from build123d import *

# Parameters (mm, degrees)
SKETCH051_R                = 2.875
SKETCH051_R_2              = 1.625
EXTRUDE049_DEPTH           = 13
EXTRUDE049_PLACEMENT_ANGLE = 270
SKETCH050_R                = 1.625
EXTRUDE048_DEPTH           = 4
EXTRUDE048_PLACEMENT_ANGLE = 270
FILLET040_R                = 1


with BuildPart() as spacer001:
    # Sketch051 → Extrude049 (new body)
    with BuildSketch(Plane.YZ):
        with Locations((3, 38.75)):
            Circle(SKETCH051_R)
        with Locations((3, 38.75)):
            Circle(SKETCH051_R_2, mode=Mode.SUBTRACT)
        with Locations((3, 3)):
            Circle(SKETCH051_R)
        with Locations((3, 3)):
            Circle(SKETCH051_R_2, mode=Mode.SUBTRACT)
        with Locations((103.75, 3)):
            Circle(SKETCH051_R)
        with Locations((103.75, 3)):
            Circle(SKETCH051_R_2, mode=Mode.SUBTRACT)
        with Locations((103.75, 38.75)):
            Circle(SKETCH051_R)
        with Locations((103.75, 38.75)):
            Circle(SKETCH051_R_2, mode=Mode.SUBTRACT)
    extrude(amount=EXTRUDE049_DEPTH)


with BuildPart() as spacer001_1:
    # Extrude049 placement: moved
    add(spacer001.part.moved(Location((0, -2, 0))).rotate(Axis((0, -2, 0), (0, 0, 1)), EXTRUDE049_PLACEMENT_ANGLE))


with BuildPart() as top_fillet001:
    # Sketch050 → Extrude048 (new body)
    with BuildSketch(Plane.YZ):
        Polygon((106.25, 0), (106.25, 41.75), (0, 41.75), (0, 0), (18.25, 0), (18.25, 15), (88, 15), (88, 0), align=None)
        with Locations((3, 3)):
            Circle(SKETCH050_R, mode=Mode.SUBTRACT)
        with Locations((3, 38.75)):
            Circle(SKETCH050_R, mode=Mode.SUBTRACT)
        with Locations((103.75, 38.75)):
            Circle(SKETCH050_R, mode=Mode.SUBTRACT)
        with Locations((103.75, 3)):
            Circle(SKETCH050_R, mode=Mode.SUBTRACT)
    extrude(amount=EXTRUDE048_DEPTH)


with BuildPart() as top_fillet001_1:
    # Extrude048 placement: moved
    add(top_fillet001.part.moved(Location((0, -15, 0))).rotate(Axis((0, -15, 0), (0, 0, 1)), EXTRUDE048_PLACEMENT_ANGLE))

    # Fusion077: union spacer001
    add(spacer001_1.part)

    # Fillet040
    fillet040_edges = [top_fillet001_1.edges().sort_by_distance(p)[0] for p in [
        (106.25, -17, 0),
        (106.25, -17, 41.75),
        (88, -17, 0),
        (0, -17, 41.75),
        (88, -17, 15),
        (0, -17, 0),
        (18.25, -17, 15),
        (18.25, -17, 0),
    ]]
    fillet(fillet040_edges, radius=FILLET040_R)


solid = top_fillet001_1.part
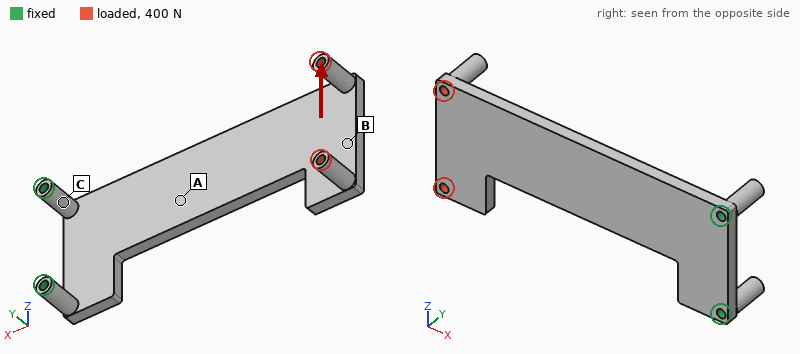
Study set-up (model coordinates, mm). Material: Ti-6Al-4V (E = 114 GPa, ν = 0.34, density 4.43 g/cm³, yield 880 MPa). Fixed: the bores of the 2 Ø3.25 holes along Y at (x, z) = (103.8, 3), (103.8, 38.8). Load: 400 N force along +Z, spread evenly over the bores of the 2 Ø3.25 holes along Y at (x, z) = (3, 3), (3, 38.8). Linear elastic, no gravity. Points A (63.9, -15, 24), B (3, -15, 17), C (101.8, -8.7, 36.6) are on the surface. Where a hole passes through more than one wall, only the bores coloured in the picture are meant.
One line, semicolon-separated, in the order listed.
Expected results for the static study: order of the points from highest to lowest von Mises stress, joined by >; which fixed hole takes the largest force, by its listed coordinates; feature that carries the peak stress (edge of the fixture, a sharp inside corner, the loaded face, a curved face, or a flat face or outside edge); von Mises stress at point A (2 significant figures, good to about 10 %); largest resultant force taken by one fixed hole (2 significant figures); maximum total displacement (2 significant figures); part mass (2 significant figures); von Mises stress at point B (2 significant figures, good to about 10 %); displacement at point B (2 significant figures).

A > B > C; (103.8, 3); a curved face; 46 MPa; 1.3 kN; 0.49 mm; 64 g; 26 MPa; 0.23 mm
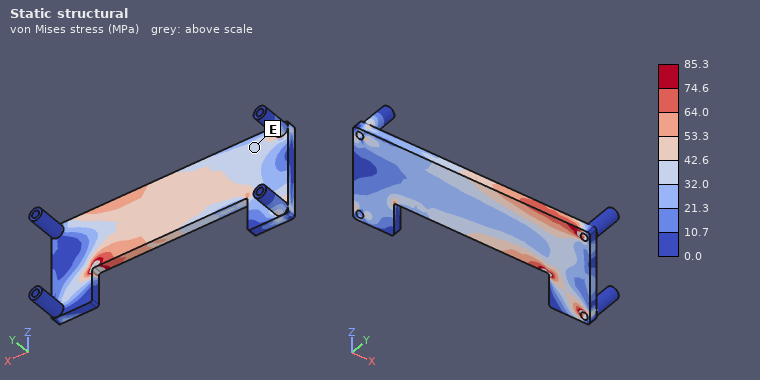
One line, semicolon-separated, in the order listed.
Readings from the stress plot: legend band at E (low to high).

32.0 to 42.6 MPa
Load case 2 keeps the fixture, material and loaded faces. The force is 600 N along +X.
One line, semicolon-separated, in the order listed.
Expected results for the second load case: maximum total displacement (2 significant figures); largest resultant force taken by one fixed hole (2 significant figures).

1.4 mm; 360 N
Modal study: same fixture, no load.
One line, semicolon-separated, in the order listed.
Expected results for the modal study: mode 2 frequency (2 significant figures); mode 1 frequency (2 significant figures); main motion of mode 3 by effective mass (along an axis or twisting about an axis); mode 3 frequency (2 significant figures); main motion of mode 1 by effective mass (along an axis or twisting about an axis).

1300 Hz; 250 Hz; along Z; 1700 Hz; along Y
